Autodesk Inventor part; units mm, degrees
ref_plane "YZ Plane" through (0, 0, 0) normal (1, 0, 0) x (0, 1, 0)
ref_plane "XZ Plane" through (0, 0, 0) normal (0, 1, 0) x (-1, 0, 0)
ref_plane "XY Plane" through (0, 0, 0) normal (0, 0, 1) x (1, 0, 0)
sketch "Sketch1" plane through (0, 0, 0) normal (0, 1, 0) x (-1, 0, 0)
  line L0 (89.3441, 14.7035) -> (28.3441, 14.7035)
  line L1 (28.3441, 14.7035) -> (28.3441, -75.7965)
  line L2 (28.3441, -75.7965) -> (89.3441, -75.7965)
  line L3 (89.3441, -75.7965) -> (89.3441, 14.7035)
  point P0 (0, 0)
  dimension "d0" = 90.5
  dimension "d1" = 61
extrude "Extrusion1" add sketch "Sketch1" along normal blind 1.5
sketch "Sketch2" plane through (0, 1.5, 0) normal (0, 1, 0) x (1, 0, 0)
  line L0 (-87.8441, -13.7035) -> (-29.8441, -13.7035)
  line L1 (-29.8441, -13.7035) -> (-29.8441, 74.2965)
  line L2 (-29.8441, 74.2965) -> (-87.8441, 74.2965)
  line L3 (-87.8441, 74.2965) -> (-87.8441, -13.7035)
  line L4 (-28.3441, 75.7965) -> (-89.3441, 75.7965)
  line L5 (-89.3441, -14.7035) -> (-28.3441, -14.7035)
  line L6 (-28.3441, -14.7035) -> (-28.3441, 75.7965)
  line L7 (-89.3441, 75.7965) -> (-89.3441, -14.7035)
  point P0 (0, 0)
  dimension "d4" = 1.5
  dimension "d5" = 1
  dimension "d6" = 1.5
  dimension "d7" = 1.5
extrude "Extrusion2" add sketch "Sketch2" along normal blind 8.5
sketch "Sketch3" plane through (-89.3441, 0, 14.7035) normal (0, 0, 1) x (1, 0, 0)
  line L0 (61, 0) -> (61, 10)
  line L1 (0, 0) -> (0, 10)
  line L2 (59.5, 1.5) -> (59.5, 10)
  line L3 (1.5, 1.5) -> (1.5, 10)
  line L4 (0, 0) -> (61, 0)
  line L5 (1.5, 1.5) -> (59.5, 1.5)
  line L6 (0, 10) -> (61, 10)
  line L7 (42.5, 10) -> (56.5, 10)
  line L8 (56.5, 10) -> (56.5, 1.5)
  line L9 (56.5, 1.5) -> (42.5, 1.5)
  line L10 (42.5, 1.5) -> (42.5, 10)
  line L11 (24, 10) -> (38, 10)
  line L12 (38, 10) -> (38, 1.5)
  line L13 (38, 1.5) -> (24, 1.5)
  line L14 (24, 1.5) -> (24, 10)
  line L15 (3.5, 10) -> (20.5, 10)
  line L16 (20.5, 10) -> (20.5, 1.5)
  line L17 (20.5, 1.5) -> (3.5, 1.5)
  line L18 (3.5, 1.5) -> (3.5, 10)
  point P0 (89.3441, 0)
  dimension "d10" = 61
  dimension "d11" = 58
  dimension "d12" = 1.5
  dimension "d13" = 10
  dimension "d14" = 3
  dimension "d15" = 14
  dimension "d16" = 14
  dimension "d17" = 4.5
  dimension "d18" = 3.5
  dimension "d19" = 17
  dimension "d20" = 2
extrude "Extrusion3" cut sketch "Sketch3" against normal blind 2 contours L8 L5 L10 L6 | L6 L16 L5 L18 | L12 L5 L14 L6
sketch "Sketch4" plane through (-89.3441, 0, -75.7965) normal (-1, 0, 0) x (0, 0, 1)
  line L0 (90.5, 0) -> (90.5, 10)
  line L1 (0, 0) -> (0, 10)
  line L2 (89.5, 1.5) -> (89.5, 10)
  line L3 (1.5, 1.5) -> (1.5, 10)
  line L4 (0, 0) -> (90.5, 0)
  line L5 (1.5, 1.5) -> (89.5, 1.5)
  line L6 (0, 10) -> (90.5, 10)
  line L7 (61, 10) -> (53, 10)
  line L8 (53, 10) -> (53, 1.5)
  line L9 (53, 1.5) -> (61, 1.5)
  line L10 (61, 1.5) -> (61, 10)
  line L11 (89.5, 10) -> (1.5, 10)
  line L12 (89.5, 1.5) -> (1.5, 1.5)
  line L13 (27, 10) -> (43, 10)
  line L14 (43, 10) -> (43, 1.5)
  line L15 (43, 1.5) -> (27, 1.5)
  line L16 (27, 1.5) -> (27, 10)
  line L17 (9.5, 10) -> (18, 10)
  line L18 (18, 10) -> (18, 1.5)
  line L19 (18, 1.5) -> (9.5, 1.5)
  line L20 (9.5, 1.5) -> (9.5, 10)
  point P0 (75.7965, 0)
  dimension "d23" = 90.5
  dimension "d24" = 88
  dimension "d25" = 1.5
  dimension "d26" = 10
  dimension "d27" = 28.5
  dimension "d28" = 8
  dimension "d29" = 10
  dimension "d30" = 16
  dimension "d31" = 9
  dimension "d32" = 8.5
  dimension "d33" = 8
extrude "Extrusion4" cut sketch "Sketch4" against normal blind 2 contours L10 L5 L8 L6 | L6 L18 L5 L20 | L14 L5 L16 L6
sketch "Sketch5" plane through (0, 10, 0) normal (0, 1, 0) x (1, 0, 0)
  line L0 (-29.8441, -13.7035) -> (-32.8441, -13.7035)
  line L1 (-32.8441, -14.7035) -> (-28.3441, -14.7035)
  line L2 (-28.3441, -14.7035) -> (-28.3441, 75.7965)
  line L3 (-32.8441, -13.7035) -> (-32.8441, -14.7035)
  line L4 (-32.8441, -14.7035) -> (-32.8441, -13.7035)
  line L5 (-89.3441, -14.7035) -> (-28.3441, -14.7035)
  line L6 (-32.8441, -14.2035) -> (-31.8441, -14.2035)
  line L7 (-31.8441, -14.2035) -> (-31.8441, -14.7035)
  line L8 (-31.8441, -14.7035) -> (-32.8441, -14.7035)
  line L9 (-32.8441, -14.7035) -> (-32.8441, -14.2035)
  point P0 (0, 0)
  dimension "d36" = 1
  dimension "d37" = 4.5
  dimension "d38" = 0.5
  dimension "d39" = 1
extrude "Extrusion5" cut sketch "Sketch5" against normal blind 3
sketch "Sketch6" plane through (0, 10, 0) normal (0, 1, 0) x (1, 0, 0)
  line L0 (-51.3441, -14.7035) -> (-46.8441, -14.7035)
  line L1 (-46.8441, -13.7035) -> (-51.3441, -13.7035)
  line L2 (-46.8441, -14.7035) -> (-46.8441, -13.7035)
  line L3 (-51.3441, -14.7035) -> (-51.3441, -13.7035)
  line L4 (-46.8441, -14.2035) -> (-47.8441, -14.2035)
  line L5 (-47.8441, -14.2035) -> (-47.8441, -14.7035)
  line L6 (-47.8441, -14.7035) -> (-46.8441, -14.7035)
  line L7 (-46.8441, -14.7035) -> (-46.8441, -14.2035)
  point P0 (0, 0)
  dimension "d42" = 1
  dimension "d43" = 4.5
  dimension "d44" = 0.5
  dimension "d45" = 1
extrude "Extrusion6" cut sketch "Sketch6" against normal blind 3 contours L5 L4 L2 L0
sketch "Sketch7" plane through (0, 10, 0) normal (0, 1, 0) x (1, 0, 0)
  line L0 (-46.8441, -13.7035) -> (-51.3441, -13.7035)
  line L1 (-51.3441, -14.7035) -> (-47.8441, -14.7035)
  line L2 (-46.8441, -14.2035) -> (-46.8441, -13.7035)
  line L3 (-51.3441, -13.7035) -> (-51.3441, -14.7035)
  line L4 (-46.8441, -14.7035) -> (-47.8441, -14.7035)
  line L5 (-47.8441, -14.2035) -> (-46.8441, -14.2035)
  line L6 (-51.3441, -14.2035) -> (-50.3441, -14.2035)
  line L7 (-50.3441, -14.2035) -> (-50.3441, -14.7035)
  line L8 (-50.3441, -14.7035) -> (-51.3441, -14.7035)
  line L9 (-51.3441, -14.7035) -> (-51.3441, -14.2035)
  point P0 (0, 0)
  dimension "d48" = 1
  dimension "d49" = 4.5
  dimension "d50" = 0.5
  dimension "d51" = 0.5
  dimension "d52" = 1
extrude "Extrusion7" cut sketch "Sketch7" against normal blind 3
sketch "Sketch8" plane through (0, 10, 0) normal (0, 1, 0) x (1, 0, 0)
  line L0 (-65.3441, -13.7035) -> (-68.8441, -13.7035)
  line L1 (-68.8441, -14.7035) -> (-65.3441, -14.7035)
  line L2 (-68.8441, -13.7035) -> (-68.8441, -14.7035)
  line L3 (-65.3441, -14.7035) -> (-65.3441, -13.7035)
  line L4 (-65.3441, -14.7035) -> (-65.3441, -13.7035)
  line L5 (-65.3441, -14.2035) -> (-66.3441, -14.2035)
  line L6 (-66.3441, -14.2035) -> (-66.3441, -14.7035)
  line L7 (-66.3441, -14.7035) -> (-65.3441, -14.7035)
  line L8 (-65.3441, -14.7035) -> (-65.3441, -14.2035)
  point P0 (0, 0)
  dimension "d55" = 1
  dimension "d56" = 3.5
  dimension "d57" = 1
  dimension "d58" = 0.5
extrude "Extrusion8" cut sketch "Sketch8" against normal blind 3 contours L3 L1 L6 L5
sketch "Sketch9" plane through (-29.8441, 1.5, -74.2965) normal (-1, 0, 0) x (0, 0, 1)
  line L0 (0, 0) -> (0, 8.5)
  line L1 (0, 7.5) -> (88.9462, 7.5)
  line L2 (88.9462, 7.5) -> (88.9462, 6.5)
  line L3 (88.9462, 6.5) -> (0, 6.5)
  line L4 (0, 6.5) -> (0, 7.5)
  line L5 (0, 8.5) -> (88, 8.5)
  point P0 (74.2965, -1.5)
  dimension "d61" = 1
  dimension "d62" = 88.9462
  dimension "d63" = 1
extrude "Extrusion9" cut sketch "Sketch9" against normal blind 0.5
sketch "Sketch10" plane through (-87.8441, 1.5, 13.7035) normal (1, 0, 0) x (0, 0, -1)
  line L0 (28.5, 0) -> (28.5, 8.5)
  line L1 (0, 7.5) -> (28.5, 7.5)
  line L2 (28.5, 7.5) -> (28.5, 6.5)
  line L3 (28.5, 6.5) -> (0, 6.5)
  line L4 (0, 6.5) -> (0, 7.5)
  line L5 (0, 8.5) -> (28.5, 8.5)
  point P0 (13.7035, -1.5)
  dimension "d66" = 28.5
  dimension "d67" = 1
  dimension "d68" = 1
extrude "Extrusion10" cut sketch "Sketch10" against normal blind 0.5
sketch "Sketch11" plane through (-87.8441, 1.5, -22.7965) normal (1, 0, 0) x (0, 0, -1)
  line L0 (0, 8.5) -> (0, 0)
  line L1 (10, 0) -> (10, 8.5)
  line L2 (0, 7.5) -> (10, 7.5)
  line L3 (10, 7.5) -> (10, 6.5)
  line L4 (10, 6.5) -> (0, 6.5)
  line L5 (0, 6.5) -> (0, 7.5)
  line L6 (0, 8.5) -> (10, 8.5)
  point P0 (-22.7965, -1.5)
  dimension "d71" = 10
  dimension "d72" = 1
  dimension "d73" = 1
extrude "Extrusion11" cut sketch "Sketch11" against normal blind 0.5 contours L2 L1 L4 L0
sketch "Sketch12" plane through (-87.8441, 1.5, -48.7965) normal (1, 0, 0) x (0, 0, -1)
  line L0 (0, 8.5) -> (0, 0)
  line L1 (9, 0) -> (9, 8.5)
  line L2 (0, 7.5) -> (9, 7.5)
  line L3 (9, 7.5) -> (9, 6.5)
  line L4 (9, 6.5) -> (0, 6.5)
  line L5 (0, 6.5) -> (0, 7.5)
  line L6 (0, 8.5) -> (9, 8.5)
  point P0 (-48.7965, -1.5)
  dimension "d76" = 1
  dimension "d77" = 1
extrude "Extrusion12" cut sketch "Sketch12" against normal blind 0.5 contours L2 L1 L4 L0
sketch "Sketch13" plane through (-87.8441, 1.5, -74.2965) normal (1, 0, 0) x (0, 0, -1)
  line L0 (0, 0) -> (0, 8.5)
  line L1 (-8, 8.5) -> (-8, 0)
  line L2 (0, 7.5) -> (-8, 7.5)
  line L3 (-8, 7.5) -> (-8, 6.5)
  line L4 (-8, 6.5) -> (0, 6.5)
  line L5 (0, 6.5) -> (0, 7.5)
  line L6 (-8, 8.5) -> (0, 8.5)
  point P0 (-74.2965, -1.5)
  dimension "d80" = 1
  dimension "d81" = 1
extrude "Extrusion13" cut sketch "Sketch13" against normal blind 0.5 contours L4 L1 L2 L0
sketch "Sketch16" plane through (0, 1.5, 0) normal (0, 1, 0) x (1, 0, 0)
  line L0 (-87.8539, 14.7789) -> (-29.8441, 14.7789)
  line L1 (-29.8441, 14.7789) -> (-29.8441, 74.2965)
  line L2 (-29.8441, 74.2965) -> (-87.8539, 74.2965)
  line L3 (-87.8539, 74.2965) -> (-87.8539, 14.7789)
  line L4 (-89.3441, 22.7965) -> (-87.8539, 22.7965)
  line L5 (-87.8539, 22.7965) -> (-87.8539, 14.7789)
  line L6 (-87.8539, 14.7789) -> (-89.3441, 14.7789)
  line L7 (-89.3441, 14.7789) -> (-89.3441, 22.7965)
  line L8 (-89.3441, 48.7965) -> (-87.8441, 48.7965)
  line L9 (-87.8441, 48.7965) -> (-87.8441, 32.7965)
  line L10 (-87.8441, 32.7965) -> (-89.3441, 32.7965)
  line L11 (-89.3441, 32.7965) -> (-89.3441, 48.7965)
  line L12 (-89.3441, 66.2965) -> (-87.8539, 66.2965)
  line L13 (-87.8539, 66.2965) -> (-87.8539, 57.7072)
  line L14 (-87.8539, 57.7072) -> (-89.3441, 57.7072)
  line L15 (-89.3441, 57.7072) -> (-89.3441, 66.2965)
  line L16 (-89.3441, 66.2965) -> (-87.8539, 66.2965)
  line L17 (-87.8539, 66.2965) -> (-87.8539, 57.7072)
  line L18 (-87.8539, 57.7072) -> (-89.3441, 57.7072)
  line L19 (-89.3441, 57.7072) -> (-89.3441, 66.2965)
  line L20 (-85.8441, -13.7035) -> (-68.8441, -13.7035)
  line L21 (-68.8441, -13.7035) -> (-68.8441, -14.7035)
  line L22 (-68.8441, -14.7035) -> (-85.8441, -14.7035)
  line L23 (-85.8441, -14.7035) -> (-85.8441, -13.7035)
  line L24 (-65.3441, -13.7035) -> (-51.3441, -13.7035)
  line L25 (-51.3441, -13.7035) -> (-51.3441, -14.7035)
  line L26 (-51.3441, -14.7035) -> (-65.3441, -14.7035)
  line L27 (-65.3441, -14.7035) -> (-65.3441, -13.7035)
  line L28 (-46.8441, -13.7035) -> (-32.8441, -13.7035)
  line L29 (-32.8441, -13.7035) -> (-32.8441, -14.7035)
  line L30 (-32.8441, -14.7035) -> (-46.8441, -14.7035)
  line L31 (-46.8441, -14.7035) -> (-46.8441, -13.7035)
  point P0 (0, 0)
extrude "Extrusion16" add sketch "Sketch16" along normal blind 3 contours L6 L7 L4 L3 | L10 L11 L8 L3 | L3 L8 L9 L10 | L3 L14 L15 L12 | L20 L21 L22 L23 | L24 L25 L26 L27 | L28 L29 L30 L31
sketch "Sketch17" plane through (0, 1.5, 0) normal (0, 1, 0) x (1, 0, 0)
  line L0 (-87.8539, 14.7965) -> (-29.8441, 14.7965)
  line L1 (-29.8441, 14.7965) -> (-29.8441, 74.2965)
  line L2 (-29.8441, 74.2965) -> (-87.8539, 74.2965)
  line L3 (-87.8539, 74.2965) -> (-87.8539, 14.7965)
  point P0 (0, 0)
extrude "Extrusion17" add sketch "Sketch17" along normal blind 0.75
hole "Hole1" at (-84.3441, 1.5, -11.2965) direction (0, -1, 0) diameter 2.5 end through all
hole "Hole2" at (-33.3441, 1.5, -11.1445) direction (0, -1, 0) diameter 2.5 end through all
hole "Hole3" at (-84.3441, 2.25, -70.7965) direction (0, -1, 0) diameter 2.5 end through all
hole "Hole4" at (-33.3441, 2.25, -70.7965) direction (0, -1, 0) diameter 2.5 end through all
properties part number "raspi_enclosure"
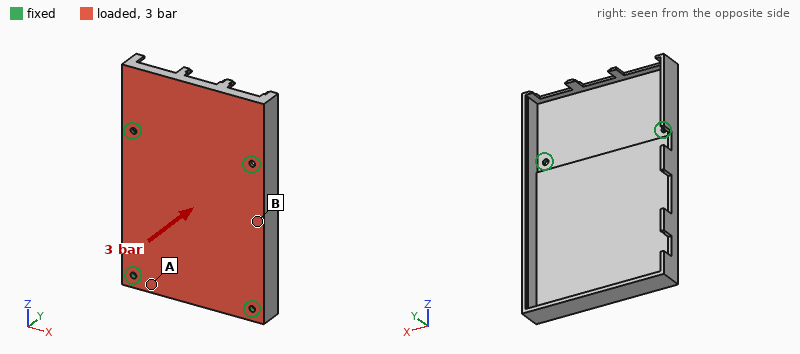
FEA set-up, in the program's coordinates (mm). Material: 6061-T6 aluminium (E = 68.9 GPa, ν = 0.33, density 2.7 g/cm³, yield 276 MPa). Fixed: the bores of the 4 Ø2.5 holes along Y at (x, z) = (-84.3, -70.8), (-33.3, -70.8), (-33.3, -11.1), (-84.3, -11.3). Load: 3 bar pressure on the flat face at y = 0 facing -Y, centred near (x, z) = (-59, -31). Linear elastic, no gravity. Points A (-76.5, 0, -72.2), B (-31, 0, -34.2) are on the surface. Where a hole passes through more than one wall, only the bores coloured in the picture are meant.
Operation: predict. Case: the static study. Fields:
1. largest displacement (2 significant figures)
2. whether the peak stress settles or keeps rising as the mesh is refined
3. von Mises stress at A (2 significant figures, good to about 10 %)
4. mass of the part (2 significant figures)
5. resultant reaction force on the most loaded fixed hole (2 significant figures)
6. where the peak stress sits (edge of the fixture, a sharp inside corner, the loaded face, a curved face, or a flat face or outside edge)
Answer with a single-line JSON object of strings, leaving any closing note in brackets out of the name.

{"largest displacement": "0.40 mm", "whether the peak stress settles or keeps rising as the mesh is refined": "keeps rising", "von Mises stress at A": "52 MPa", "mass of the part": "37 g", "resultant reaction force on the most loaded fixed hole": "550 N", "where the peak stress sits": "edge of the fixture"}
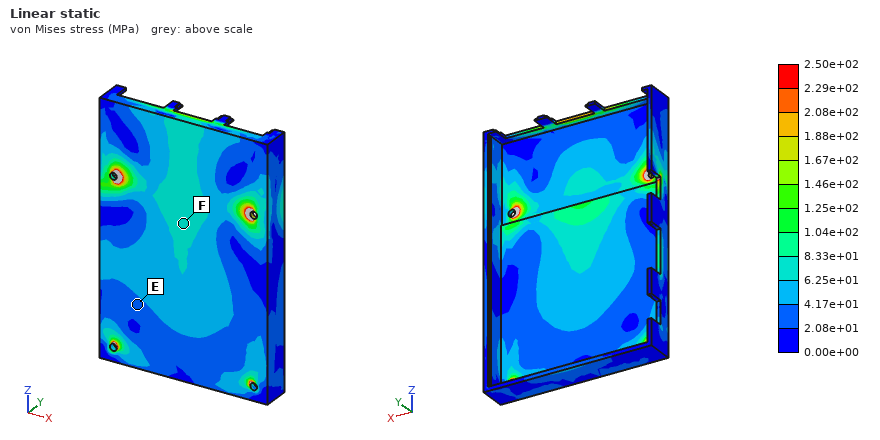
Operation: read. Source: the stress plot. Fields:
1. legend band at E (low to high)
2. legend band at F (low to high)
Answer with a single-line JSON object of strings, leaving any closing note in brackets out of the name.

{"legend band at E": "2.08e+01 to 4.17e+01 MPa", "legend band at F": "6.25e+01 to 8.33e+01 MPa"}
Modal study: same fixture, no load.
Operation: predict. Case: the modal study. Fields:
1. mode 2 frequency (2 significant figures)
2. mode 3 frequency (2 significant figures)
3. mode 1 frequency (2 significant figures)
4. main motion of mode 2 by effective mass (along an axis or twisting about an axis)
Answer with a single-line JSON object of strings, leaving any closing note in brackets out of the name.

{"mode 2 frequency": "2500 Hz", "mode 3 frequency": "3800 Hz", "mode 1 frequency": "2200 Hz", "main motion of mode 2 by effective mass": "along Y"}
